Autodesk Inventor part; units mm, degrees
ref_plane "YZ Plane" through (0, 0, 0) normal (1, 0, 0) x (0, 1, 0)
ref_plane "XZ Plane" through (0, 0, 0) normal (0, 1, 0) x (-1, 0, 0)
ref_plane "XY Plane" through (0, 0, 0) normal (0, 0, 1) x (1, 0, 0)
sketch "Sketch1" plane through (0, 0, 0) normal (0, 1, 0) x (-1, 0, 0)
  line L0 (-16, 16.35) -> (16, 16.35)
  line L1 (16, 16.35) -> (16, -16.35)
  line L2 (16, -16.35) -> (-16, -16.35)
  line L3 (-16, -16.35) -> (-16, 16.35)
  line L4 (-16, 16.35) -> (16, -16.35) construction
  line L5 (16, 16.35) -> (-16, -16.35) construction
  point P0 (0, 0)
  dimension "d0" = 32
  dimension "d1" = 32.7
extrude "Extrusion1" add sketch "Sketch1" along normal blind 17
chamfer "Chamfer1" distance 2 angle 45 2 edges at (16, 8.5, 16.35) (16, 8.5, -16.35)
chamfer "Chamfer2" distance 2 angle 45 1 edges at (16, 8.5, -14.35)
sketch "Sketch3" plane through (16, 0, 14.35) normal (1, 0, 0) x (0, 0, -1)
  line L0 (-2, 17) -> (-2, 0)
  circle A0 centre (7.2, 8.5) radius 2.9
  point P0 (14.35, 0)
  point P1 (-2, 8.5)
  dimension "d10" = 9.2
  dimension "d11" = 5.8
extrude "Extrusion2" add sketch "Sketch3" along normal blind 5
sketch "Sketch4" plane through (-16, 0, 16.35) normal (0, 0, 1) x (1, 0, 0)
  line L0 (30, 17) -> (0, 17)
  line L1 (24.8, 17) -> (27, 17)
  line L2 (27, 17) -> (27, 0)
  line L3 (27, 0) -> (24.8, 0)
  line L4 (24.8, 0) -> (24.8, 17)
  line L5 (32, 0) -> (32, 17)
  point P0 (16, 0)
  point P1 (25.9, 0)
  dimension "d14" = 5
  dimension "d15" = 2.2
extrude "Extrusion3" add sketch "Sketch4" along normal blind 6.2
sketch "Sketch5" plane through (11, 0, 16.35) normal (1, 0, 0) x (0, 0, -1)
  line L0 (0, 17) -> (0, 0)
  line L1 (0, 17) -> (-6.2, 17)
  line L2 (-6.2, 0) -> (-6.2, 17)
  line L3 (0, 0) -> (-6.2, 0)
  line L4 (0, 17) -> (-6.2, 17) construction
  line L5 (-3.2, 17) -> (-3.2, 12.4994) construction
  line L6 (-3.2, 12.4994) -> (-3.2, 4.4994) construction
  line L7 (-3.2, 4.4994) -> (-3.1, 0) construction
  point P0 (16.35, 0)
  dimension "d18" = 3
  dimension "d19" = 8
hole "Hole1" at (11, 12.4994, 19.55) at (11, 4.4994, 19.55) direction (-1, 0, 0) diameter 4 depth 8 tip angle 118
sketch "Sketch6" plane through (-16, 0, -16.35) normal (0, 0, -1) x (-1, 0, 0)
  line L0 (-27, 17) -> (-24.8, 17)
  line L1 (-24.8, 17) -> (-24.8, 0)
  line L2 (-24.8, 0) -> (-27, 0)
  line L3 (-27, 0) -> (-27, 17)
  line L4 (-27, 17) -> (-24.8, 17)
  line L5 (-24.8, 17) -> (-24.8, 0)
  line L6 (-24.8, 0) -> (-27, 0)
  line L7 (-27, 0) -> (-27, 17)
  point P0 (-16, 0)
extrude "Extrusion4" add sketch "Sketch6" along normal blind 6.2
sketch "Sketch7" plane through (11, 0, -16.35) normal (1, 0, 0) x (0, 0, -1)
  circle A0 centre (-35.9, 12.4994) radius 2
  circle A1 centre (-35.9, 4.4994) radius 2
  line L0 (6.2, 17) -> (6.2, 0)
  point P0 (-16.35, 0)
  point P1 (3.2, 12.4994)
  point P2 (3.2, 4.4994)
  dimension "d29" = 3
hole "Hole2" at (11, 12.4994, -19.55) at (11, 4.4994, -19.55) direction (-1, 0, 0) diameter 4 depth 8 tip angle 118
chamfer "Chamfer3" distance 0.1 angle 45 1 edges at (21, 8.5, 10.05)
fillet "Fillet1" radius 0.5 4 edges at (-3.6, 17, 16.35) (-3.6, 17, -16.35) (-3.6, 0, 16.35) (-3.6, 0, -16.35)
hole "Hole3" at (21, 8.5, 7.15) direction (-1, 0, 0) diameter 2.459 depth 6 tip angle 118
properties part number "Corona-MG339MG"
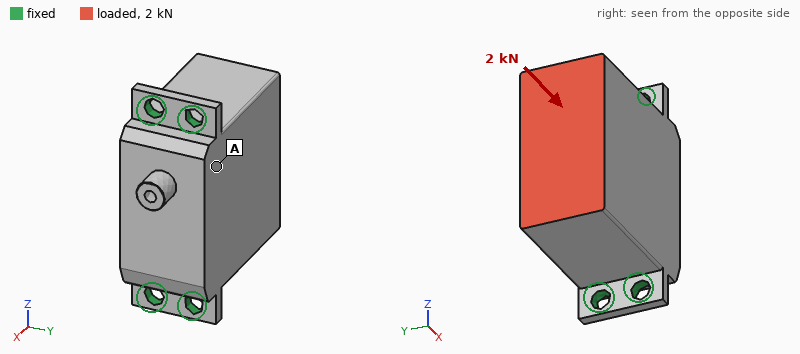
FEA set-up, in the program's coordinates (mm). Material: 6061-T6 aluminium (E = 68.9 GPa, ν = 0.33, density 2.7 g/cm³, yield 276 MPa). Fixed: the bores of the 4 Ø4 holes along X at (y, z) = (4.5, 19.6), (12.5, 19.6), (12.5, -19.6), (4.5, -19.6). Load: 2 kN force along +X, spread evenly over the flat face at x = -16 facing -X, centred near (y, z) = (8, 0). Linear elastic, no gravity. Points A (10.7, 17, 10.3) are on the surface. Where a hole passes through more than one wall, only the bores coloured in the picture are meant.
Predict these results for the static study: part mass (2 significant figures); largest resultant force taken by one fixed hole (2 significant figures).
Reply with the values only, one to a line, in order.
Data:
49 g
510 N
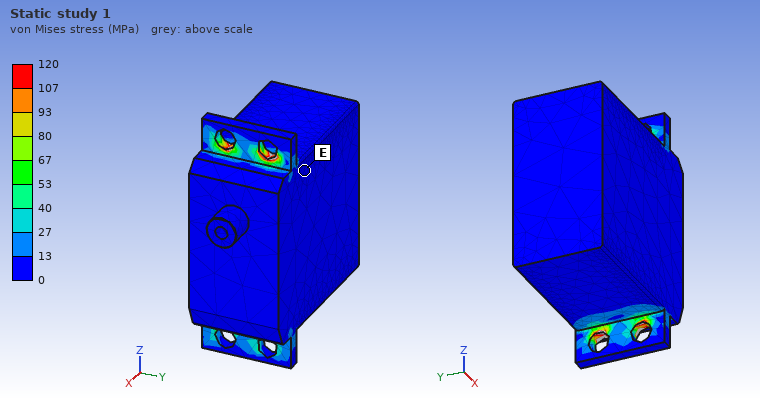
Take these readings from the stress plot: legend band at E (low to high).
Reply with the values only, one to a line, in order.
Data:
0 to 13 MPa
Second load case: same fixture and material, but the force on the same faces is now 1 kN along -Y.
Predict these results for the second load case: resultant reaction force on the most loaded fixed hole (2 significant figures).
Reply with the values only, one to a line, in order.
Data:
1.3 kN
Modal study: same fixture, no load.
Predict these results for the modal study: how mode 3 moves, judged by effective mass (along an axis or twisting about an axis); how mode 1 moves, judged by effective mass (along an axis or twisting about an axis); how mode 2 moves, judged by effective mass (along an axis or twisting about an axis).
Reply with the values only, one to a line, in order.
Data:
along X
along Y
along Z
